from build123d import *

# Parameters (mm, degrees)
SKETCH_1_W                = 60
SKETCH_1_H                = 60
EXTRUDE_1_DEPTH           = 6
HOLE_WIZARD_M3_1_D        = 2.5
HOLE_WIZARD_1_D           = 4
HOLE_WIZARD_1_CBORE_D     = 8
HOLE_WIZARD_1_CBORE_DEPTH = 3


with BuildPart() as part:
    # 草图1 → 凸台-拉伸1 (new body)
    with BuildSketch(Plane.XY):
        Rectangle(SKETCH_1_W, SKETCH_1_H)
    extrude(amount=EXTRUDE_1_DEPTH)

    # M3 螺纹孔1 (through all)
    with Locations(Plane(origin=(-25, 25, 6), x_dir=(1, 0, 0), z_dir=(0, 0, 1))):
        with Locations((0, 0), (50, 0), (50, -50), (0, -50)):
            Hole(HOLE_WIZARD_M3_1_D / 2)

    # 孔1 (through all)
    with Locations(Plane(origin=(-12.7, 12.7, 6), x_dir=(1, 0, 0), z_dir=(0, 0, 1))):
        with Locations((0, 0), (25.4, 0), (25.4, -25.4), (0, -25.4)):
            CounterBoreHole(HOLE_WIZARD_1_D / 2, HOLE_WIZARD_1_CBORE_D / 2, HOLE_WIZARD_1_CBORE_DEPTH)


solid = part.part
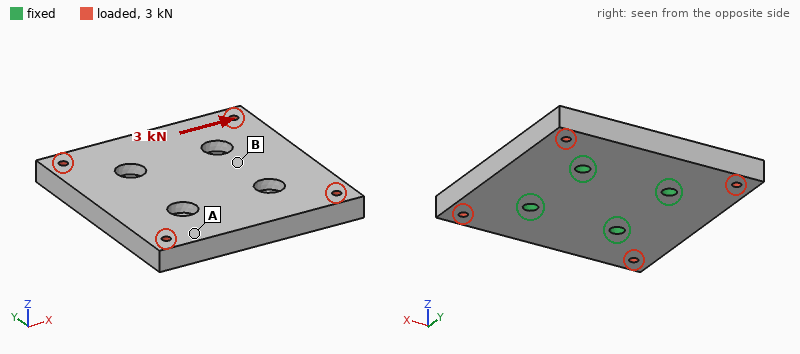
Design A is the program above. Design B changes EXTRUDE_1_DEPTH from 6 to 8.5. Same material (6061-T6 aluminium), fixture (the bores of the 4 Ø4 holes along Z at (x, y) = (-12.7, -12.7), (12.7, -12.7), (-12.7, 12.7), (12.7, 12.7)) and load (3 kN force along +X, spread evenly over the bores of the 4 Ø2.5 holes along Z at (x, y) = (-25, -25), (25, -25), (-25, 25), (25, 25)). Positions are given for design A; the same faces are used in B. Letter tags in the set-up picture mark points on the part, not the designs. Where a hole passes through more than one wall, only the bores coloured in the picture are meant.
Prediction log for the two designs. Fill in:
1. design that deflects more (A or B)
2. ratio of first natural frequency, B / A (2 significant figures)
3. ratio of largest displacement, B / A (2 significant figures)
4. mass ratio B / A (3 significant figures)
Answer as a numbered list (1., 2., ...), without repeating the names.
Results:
1. A
2. 1.1
3. 0.86
4. 1.41
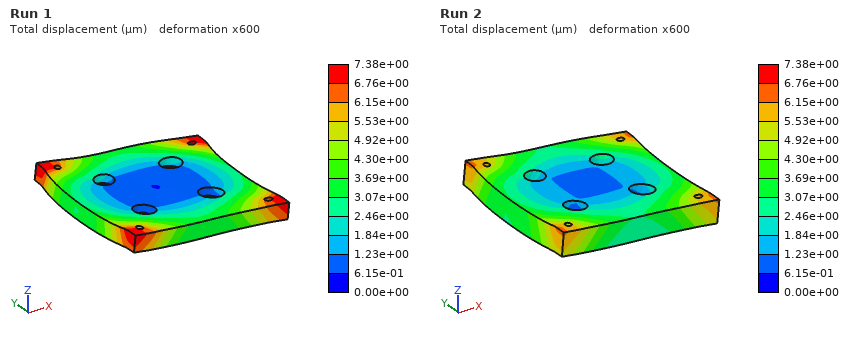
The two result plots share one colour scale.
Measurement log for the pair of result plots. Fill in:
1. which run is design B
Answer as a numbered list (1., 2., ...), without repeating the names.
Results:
1. Run 2
